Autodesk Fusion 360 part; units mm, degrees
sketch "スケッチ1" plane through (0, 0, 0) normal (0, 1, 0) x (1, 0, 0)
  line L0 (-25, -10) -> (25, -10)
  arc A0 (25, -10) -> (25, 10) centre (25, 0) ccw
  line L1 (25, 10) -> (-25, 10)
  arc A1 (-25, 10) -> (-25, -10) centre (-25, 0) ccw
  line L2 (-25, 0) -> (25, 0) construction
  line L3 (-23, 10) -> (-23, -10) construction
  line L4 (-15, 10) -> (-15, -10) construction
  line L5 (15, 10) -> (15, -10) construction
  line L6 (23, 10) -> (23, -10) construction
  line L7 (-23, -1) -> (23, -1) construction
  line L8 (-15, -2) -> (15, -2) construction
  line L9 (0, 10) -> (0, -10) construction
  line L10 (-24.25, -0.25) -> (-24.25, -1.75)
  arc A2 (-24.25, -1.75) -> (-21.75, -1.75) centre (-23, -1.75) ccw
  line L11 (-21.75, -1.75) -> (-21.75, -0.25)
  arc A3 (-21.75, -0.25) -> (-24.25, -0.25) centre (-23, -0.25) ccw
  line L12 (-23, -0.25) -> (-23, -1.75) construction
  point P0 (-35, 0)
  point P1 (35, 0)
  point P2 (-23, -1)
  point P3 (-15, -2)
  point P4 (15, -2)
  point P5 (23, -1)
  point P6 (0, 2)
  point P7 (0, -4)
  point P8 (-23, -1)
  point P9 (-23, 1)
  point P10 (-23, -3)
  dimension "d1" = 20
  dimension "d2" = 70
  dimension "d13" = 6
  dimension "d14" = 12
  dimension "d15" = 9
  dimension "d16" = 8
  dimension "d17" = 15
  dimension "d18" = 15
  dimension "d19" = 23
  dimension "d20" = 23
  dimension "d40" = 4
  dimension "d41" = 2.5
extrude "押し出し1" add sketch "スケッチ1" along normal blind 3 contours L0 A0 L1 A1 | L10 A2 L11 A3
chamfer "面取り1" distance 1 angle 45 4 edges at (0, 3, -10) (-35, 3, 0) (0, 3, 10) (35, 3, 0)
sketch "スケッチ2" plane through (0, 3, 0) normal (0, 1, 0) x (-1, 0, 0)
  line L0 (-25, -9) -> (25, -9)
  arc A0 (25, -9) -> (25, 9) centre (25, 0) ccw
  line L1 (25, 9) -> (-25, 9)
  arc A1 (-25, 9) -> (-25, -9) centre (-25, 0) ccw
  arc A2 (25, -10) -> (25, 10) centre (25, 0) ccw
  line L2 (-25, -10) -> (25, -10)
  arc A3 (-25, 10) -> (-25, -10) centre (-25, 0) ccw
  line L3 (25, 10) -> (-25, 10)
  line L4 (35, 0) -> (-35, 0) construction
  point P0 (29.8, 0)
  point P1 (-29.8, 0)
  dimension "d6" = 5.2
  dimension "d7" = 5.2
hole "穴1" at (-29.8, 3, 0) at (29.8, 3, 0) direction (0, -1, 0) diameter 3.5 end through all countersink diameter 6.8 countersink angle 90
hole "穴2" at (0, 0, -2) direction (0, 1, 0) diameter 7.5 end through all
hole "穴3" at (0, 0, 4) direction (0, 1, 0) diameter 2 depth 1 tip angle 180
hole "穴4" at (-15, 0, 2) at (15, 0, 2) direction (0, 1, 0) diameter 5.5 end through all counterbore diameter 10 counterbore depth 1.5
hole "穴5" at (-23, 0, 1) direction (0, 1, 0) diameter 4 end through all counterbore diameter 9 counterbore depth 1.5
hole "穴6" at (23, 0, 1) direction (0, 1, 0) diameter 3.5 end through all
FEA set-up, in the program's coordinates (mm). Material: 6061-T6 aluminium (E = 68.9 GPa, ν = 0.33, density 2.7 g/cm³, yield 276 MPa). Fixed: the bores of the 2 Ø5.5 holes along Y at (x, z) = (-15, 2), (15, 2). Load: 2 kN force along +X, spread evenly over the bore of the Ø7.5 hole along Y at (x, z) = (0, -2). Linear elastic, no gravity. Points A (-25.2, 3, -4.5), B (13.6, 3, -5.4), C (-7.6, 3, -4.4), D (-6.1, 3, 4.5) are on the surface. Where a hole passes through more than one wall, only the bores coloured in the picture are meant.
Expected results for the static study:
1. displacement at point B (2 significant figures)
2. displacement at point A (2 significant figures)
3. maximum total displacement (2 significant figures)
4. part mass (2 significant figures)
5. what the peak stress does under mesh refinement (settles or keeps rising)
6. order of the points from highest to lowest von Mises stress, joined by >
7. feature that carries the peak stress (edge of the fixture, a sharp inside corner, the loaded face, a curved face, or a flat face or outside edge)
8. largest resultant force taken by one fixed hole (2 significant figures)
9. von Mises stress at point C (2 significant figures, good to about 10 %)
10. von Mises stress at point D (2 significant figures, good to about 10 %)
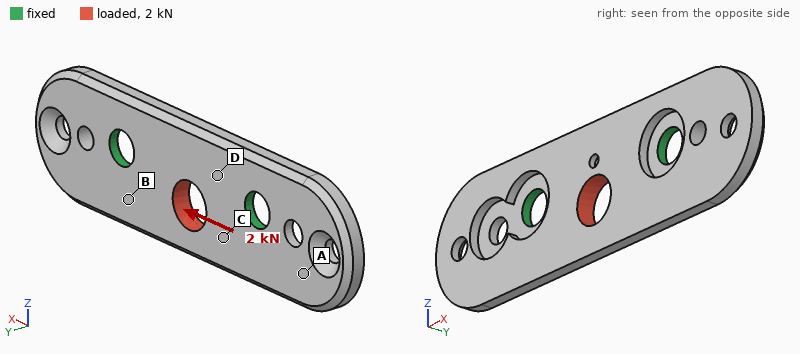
4.6 µm
6.4 µm
15 µm
8.6 g
keeps rising
C > D > B > A
edge of the fixture
1.0 kN
37 MPa
26 MPa
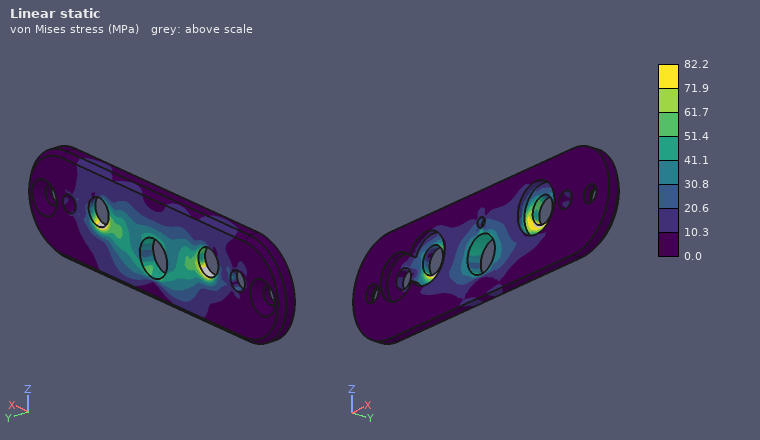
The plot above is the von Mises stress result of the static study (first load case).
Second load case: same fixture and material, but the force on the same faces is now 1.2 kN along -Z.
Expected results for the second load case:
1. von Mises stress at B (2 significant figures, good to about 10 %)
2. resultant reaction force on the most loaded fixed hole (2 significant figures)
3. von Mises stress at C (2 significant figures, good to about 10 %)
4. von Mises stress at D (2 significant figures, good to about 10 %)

13 MPa
610 N
25 MPa
14 MPa
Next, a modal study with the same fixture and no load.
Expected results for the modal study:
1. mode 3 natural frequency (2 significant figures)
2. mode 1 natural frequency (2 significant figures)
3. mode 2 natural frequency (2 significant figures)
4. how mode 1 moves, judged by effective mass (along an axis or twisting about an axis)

8700 Hz
5700 Hz
6000 Hz
along Y
